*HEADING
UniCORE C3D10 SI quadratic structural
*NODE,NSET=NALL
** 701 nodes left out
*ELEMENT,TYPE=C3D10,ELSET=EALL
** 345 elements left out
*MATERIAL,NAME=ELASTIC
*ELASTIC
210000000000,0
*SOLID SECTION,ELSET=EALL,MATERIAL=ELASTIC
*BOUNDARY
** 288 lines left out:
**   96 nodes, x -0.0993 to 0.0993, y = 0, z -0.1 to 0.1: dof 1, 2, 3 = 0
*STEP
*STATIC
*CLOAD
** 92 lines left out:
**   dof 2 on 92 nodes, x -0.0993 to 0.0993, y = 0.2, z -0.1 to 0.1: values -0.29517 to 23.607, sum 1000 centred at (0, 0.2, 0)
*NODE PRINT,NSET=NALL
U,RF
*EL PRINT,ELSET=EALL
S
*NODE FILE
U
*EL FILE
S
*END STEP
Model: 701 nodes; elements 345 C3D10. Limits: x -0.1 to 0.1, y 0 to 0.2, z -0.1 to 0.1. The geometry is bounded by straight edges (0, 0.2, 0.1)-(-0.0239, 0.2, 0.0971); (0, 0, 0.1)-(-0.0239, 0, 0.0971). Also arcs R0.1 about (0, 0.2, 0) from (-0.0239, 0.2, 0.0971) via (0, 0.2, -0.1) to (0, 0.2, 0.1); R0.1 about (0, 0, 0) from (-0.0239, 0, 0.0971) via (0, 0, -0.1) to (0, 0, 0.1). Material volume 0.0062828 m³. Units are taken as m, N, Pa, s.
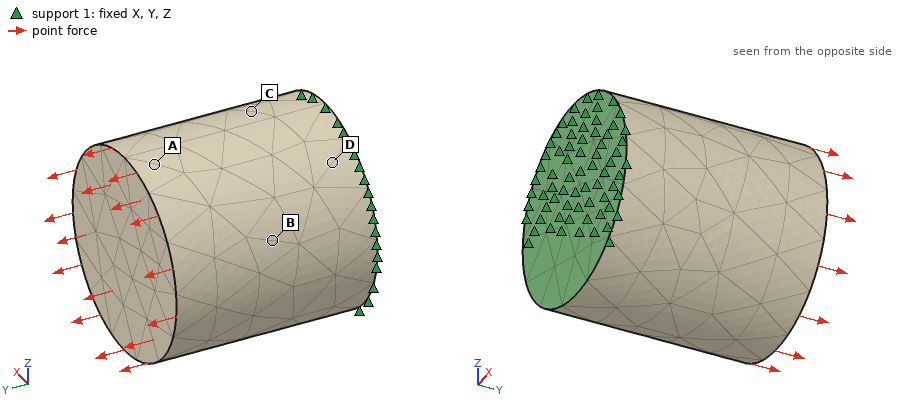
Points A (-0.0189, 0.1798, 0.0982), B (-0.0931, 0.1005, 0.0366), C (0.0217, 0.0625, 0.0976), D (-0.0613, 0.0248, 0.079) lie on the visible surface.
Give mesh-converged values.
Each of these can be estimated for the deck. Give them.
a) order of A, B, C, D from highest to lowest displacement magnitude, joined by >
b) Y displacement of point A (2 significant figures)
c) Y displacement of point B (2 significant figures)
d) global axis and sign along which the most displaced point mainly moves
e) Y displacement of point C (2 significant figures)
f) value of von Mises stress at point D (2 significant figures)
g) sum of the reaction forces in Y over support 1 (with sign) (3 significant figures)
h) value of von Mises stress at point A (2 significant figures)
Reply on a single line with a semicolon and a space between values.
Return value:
A > B > C > D; 2.7e-08 m; 1.5e-08 m; +Y; 9.5e-09 m; 32000 Pa; -1000 N; 33000 Pa
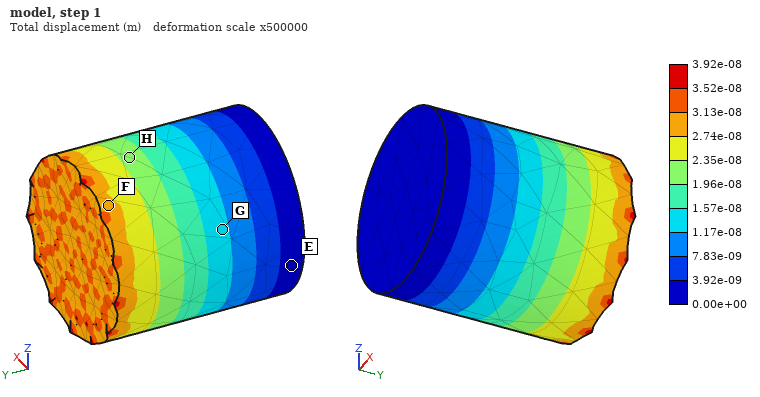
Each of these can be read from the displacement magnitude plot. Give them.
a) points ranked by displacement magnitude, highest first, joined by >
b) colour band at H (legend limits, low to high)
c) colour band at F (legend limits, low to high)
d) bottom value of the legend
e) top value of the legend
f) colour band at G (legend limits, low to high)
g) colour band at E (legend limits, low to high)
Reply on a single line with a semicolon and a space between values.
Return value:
F > H > G > E; 1.96e-08 to 2.35e-08 m; 2.74e-08 to 3.13e-08 m; 0.00e+00 m; 3.92e-08 m; 1.17e-08 to 1.57e-08 m; 0.00e+00 to 3.92e-09 m
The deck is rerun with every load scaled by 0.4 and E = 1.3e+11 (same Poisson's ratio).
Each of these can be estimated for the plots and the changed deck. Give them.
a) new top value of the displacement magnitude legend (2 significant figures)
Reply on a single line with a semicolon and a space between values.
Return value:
2.5e-08 m
